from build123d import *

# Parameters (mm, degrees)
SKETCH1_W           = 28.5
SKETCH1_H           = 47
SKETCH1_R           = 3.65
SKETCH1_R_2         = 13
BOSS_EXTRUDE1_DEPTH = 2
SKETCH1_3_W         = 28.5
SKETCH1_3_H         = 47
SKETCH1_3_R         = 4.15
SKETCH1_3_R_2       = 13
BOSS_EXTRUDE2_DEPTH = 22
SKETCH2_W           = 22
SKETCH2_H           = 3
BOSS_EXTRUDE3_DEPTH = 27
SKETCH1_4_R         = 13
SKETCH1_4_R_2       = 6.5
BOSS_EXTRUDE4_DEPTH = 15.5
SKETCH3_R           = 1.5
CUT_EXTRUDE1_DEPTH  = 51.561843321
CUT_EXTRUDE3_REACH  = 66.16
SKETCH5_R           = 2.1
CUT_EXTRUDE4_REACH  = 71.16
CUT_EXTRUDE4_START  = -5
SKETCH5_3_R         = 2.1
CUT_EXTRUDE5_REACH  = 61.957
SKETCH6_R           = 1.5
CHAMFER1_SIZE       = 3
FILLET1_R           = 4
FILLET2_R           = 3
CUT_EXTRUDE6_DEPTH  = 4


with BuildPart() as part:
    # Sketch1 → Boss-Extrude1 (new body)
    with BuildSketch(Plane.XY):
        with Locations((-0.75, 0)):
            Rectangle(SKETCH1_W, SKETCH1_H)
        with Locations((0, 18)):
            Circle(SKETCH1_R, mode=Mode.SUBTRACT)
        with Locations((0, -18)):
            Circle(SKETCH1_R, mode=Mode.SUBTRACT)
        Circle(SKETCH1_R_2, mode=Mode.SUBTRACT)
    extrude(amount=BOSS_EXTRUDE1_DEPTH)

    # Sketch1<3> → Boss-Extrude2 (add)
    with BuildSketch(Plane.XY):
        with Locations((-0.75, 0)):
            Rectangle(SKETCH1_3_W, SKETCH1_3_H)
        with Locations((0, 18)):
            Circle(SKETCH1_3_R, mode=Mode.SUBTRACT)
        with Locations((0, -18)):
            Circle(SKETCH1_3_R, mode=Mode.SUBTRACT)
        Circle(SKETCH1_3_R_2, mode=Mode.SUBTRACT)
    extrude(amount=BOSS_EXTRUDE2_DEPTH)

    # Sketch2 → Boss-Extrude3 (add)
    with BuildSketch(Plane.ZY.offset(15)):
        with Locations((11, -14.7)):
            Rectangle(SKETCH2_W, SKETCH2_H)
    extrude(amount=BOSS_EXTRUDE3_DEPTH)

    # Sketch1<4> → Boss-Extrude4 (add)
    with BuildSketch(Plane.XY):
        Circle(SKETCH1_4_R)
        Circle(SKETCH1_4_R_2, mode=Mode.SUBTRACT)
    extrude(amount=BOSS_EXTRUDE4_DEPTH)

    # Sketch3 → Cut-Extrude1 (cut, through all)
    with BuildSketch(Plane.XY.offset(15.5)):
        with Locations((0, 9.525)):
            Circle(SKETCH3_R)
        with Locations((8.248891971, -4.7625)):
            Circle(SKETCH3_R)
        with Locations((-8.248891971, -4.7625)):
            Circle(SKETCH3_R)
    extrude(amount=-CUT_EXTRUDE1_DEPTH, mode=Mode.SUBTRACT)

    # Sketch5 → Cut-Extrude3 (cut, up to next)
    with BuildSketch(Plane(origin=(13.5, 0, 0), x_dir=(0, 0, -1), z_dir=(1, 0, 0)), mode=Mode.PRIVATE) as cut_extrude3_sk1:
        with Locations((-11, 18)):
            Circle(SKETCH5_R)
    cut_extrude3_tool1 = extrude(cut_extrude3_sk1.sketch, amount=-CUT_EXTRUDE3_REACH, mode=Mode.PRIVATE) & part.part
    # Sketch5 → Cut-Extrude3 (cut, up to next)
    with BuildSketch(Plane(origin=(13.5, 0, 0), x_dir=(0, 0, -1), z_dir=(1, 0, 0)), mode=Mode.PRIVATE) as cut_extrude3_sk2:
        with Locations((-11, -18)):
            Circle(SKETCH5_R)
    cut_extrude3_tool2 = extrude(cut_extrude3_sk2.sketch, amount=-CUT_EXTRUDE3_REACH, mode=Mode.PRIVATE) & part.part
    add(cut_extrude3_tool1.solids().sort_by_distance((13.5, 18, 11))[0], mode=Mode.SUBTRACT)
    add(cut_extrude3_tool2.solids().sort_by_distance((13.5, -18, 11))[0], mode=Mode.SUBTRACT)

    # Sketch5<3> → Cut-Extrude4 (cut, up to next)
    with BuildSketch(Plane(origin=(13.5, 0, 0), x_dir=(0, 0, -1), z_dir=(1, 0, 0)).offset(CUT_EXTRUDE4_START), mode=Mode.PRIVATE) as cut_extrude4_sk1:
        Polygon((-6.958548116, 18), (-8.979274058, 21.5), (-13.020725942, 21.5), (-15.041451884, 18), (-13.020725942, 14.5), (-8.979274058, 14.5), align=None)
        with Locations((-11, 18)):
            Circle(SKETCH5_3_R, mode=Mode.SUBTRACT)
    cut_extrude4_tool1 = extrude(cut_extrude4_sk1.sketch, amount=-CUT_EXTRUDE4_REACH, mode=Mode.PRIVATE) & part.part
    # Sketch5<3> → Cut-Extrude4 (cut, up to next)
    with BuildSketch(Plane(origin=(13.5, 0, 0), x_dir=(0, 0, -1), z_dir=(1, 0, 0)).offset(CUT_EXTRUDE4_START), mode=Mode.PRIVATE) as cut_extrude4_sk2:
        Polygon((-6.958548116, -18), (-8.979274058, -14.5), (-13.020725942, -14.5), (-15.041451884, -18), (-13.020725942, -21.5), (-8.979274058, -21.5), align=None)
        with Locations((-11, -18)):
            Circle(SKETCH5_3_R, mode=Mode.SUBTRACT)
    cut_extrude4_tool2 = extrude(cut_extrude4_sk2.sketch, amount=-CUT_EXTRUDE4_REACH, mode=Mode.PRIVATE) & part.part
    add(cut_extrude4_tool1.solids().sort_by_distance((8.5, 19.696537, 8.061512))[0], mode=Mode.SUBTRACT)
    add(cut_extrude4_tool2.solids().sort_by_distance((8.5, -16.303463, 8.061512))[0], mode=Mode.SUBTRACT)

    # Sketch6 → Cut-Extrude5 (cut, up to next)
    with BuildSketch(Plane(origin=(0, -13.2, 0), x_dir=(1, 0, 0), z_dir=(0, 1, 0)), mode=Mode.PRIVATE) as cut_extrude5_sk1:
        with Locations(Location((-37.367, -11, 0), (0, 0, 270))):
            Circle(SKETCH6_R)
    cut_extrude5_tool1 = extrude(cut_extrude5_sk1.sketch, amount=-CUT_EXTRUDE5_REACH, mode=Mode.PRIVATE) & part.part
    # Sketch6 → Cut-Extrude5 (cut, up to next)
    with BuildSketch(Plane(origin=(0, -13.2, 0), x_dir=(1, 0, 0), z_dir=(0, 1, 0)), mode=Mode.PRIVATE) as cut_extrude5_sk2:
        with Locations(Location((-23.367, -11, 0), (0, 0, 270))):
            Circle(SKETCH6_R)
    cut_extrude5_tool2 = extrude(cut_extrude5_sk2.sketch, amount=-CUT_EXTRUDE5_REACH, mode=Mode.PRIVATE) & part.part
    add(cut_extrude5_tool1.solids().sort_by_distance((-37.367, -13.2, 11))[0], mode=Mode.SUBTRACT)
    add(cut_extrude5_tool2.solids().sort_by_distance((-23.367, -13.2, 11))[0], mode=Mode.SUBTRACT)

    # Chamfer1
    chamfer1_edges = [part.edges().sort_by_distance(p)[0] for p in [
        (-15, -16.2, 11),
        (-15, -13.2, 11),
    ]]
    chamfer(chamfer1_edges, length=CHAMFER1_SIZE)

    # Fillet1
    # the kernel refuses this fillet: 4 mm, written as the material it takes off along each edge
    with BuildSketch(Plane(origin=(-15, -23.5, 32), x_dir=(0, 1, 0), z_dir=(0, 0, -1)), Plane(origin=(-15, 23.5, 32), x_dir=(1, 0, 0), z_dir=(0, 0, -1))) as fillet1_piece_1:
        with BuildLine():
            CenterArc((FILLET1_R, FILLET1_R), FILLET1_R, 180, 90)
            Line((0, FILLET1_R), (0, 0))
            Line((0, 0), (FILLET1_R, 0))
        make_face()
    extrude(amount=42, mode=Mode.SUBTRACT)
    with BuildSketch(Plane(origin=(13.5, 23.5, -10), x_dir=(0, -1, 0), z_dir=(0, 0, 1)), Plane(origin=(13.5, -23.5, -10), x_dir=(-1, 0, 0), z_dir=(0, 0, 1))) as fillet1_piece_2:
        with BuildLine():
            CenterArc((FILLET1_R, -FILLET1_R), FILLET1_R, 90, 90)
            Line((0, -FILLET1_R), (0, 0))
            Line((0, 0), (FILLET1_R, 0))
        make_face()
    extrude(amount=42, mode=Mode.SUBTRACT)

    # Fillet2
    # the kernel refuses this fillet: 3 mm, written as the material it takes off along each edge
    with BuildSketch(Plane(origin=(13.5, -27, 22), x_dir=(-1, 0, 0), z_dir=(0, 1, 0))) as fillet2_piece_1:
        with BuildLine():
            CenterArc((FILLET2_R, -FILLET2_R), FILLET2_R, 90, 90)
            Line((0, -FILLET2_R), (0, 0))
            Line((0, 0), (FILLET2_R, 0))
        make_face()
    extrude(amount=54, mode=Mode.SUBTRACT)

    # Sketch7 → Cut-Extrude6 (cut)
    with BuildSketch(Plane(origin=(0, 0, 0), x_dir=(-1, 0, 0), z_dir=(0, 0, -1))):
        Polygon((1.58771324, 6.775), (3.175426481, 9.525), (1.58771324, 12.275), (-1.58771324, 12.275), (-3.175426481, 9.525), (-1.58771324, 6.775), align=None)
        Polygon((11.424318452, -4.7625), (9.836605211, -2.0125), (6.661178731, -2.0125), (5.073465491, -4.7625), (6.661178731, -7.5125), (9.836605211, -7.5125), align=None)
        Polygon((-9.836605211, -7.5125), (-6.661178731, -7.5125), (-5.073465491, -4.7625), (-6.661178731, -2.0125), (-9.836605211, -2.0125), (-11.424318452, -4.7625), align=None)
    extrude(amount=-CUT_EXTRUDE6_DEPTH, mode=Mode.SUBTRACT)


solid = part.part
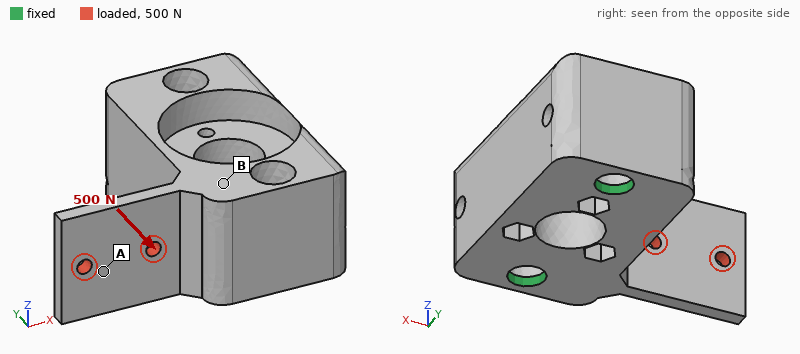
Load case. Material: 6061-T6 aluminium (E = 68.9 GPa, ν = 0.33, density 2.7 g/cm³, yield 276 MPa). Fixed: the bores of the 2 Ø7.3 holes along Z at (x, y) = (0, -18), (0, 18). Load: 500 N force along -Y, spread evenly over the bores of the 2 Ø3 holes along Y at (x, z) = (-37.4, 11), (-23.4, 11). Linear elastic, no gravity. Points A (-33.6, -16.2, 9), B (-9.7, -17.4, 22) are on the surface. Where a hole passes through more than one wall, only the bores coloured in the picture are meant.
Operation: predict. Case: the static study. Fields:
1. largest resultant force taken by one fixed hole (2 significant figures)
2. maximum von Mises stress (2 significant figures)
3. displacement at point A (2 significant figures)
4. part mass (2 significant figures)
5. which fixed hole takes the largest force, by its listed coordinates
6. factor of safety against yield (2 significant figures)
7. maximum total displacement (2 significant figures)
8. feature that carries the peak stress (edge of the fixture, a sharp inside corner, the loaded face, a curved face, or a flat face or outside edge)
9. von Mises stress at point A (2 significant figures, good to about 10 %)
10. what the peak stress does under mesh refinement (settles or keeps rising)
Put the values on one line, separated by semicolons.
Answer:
480 N; 200 MPa; 0.20 mm; 60 g; (0, 18); 1.4; 0.35 mm; the loaded face; 45 MPa; settles
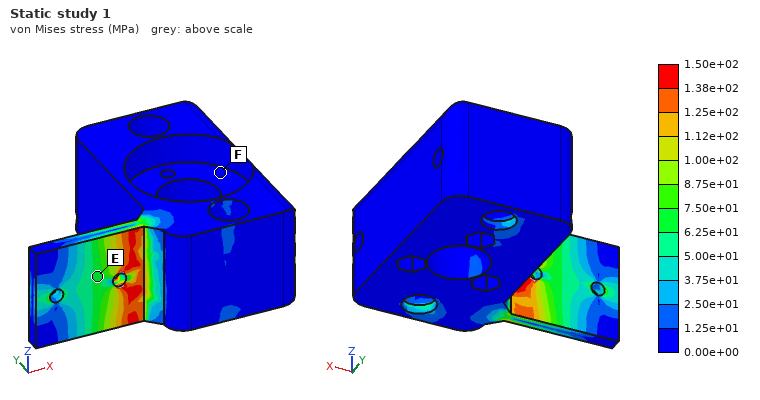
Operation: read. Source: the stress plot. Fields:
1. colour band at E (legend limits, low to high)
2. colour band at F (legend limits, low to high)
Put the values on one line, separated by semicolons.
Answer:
6.25e+01 to 7.50e+01 MPa; 0.00e+00 to 1.25e+01 MPa
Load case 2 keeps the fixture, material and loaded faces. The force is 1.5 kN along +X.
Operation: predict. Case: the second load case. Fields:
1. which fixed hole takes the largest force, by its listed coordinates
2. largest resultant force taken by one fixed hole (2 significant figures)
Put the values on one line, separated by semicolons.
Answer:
(0, -18); 1.3 kN
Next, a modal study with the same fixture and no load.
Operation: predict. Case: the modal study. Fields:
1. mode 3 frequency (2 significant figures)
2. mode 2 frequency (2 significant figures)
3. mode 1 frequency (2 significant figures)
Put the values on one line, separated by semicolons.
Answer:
9600 Hz; 3800 Hz; 3800 Hz
